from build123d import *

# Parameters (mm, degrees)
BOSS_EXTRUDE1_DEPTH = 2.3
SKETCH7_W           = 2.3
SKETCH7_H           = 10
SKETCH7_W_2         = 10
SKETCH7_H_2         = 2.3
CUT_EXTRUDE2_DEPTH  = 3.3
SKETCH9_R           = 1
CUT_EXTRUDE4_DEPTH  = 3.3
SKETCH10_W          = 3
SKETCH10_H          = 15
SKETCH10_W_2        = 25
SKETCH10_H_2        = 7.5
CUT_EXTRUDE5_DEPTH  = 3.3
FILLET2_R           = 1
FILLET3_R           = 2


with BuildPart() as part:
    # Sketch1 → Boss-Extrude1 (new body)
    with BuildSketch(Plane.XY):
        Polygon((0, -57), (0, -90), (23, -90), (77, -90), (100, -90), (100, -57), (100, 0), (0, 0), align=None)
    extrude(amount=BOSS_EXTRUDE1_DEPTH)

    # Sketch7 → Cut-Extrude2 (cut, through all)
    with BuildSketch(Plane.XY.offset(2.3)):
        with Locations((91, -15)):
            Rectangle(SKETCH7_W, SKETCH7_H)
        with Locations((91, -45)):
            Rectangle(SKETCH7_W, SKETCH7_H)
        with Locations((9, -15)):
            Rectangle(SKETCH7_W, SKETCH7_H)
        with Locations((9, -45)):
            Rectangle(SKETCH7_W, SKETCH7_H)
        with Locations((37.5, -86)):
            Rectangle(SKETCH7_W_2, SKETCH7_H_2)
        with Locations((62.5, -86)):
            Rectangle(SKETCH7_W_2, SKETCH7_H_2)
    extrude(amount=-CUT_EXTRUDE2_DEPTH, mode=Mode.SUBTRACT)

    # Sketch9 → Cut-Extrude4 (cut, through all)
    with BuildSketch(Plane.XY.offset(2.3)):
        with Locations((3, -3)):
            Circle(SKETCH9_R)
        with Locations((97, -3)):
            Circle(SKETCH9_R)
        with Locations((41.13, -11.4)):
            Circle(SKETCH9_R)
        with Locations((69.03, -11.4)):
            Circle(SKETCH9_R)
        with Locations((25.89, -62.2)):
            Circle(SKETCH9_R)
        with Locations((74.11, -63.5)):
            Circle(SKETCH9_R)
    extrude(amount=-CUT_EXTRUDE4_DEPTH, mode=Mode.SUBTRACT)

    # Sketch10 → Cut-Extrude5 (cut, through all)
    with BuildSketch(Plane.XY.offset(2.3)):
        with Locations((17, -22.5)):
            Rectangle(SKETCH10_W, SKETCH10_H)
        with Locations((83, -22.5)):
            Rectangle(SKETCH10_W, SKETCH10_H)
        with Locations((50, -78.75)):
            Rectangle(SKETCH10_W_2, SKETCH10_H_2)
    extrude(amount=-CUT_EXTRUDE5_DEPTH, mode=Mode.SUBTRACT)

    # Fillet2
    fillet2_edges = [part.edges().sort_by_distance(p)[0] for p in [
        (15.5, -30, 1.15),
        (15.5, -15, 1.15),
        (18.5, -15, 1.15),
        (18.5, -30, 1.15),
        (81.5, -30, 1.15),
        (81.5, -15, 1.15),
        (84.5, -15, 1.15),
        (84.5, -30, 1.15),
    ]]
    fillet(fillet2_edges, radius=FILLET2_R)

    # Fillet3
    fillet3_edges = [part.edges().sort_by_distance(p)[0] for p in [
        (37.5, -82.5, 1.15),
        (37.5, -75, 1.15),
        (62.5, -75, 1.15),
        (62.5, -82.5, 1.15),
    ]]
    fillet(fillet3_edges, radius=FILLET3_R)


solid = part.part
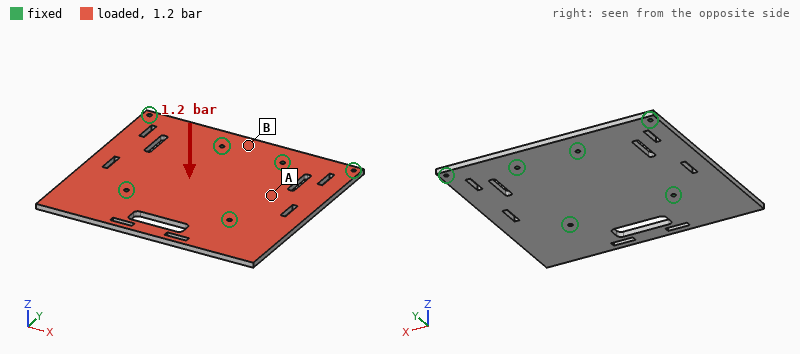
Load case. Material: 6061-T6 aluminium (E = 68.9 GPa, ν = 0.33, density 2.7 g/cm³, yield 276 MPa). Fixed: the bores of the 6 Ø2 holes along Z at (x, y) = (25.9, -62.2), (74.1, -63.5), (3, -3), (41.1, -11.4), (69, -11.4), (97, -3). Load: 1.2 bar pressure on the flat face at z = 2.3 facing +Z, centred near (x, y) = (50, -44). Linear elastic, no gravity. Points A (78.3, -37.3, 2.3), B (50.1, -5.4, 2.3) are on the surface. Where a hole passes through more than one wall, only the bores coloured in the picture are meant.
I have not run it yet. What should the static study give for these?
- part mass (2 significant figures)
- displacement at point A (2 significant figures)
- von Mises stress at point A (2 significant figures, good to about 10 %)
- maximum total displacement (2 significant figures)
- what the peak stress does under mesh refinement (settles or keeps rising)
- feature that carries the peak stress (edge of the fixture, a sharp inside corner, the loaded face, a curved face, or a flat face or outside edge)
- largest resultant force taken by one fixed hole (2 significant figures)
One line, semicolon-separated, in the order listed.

53 g; 0.053 mm; 19 MPa; 0.25 mm; keeps rising; edge of the fixture; 320 N
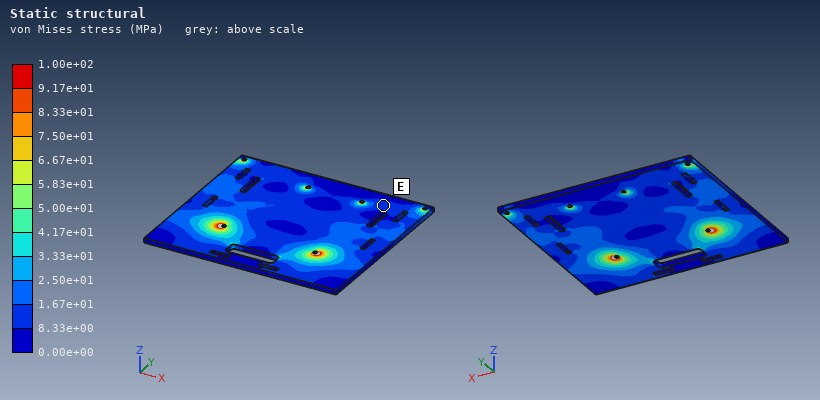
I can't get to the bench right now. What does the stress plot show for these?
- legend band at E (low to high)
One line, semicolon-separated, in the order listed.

8.33e+00 to 1.67e+01 MPa
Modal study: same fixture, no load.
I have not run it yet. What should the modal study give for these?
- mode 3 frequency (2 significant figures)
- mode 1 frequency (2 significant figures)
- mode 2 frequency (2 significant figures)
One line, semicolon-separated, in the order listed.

2100 Hz; 1800 Hz; 2000 Hz
